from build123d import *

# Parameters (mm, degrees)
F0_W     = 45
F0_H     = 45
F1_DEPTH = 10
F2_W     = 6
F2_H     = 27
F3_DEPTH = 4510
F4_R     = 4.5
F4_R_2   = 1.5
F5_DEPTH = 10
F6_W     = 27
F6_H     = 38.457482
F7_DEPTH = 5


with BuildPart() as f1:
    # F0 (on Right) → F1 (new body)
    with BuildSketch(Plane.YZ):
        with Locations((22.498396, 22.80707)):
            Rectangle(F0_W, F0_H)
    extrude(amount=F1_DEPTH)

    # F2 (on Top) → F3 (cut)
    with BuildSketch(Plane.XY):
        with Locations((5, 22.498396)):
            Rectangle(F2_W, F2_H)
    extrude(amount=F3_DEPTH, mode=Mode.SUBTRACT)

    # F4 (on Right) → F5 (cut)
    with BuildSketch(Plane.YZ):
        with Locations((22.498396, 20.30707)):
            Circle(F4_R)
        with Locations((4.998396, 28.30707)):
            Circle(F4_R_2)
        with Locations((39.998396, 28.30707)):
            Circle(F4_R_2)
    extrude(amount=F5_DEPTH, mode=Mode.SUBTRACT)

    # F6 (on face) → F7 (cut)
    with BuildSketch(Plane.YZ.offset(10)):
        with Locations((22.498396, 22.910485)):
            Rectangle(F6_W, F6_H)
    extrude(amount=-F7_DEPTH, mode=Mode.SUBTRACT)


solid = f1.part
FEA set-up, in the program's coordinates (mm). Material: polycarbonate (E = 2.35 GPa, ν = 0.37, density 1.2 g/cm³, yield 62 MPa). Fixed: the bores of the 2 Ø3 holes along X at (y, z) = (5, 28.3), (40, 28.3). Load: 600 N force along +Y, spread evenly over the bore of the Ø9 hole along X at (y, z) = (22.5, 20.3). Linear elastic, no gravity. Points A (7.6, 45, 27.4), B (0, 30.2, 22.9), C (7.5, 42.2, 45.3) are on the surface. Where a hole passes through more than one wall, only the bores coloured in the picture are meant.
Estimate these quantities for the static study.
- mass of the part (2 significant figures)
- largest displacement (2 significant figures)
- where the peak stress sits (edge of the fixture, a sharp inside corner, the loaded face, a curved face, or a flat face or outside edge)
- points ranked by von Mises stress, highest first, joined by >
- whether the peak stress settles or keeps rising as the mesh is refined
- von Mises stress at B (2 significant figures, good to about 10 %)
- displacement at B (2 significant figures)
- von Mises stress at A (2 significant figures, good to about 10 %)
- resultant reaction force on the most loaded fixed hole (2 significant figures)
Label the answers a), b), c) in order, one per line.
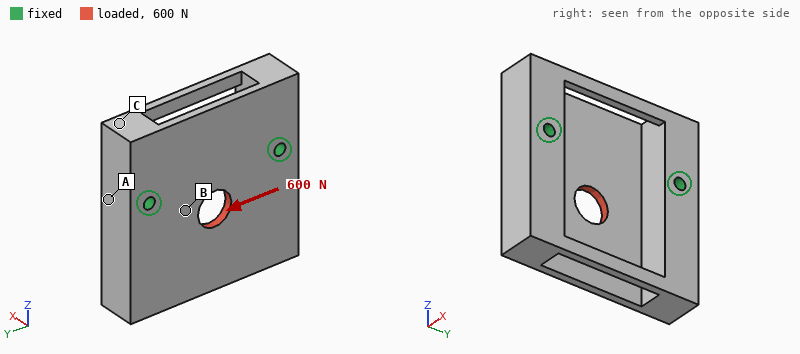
a) 13 g
b) 0.12 mm
c) edge of the fixture
d) B > A > C
e) keeps rising
f) 11 MPa
g) 0.061 mm
h) 4.1 MPa
i) 320 N
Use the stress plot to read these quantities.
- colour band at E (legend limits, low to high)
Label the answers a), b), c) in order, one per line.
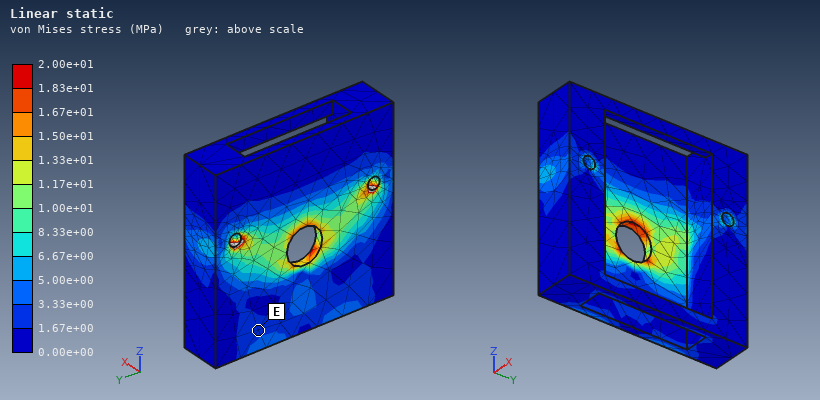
a) 1.67e+00 to 3.33e+00 MPa
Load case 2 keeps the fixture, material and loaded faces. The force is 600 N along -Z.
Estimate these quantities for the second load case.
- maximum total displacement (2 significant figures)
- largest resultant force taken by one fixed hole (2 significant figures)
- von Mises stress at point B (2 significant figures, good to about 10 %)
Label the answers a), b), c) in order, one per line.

a) 0.12 mm
b) 300 N
c) 8.5 MPa
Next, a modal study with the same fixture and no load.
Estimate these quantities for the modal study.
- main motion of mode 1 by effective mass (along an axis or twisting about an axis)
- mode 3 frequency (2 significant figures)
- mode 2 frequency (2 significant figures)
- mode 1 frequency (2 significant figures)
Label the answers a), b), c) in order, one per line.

a) along X
b) 3200 Hz
c) 2600 Hz
d) 2200 Hz
